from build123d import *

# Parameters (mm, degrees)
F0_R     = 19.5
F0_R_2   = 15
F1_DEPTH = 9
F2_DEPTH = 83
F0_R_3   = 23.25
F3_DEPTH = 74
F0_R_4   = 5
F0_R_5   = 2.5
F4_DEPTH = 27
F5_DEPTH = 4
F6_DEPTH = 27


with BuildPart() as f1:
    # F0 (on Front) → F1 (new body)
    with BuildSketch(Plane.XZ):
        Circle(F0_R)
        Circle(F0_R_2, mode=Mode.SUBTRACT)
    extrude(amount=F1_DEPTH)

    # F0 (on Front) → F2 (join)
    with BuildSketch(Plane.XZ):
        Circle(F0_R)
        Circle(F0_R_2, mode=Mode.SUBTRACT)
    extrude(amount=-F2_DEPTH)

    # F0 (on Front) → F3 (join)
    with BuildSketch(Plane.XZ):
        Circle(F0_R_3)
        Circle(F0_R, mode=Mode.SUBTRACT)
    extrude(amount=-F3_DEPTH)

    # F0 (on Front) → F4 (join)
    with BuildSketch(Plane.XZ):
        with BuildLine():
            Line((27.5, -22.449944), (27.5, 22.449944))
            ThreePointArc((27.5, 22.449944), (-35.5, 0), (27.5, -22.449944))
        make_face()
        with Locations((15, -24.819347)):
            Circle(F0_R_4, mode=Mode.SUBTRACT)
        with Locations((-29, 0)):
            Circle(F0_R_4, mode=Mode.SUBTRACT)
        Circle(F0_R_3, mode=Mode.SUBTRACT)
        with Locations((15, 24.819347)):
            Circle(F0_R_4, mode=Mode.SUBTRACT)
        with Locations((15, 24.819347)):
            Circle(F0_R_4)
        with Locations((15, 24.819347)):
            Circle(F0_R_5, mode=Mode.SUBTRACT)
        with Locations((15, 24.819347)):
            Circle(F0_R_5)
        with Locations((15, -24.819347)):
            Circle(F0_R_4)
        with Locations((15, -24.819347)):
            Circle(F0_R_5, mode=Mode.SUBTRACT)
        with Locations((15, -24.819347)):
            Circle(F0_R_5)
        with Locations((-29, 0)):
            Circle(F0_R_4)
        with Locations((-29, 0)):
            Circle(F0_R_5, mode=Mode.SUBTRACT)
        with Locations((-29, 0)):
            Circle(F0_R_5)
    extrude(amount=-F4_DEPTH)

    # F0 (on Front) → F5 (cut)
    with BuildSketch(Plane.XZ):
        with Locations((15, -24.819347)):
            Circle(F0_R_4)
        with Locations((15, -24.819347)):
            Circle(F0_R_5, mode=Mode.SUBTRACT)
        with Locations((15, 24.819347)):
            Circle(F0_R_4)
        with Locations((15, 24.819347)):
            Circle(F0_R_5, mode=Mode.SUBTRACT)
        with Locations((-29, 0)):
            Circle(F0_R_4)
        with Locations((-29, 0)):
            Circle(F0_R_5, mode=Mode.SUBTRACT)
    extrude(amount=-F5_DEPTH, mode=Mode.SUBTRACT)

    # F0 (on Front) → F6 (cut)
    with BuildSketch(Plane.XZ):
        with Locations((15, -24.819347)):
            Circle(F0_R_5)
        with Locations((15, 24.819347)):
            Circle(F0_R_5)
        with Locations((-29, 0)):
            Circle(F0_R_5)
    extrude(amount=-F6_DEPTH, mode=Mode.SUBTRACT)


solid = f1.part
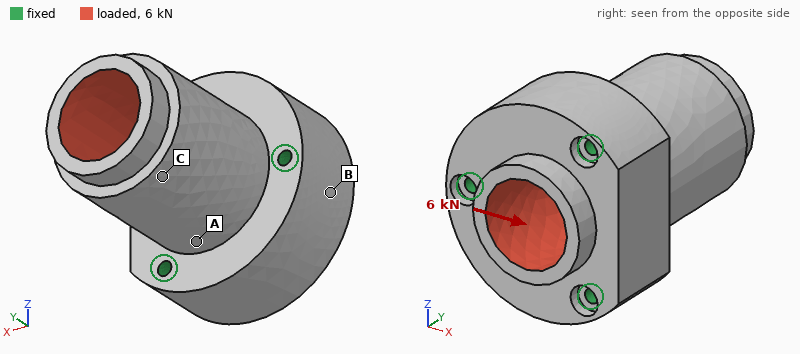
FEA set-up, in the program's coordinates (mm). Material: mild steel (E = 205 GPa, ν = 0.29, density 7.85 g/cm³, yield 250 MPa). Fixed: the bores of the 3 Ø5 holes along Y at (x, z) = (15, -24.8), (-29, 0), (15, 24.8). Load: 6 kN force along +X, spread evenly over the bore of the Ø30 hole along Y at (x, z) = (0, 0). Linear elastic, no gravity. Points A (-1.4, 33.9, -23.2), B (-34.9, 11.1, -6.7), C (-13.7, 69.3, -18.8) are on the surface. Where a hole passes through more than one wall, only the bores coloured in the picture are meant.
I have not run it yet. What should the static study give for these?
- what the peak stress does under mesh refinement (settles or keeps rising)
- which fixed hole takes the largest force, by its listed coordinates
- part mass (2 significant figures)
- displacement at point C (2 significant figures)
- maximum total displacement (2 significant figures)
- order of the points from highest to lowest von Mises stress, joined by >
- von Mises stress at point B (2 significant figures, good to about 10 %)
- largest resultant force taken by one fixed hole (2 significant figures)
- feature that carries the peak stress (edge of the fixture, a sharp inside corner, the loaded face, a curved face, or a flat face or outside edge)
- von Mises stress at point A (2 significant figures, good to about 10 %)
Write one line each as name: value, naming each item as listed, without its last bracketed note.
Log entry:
what the peak stress does under mesh refinement: keeps rising
which fixed hole takes the largest force, by its listed coordinates: (-29, 0)
part mass: 1.1 kg
displacement at point C: 6.2 µm
maximum total displacement: 8.1 µm
order of the points from highest to lowest von Mises stress, joined by >: A > B > C
von Mises stress at point B: 4.2 MPa
largest resultant force taken by one fixed hole: 3.1 kN
feature that carries the peak stress: edge of the fixture
von Mises stress at point A: 7.6 MPa
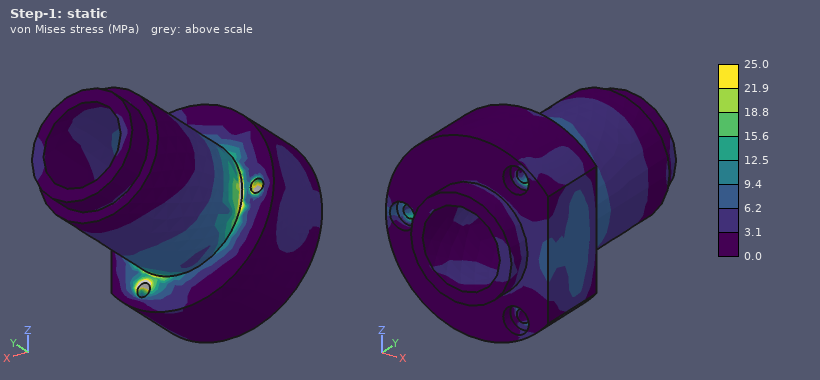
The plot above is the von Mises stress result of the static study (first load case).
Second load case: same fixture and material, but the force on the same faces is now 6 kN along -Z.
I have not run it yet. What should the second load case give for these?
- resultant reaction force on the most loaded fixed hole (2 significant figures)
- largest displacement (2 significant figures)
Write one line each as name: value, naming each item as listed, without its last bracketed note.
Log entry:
resultant reaction force on the most loaded fixed hole: 2.8 kN
largest displacement: 7.9 µm
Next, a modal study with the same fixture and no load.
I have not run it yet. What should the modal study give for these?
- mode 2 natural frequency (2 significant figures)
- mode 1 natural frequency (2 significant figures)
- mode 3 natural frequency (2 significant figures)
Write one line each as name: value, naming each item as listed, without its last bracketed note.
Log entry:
mode 2 natural frequency: 6700 Hz
mode 1 natural frequency: 6700 Hz
mode 3 natural frequency: 14 kHz
